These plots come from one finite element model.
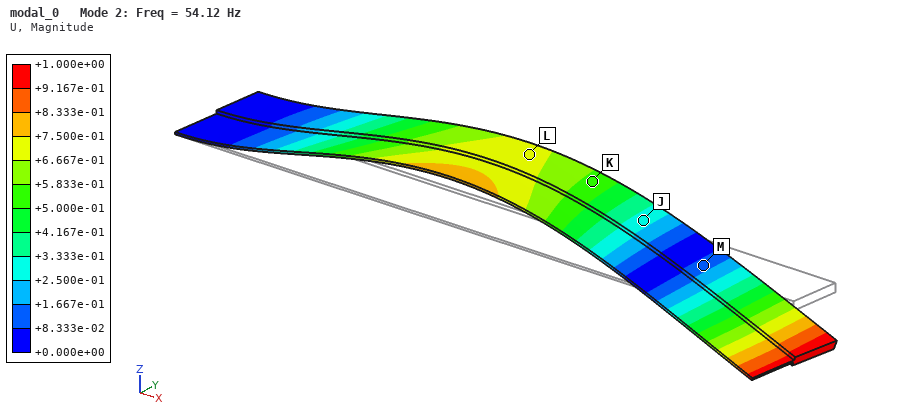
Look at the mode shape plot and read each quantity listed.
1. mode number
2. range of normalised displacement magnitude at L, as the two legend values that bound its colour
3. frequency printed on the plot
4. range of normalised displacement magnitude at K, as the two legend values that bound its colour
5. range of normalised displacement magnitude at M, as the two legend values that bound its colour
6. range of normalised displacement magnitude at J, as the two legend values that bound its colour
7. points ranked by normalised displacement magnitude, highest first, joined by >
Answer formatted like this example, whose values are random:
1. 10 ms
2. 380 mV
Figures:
1. 2
2. +6.667e-01 to +7.500e-01
3. 54.12 Hz
4. +5.000e-01 to +5.833e-01
5. +8.333e-02 to +1.667e-01
6. +2.500e-01 to +3.333e-01
7. L > K > J > M
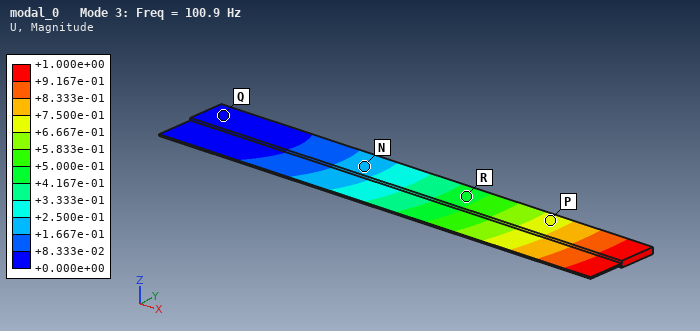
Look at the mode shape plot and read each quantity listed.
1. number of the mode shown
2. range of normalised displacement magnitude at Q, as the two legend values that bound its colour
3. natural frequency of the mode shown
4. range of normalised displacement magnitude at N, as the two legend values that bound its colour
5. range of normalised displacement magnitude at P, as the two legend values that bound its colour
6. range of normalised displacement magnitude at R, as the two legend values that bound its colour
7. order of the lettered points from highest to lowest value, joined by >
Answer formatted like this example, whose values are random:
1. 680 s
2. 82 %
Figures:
1. 3
2. +0.000e+00 to +8.333e-02
3. 100.9 Hz
4. +1.667e-01 to +2.500e-01
5. +6.667e-01 to +7.500e-01
6. +4.167e-01 to +5.000e-01
7. P > R > N > Q
